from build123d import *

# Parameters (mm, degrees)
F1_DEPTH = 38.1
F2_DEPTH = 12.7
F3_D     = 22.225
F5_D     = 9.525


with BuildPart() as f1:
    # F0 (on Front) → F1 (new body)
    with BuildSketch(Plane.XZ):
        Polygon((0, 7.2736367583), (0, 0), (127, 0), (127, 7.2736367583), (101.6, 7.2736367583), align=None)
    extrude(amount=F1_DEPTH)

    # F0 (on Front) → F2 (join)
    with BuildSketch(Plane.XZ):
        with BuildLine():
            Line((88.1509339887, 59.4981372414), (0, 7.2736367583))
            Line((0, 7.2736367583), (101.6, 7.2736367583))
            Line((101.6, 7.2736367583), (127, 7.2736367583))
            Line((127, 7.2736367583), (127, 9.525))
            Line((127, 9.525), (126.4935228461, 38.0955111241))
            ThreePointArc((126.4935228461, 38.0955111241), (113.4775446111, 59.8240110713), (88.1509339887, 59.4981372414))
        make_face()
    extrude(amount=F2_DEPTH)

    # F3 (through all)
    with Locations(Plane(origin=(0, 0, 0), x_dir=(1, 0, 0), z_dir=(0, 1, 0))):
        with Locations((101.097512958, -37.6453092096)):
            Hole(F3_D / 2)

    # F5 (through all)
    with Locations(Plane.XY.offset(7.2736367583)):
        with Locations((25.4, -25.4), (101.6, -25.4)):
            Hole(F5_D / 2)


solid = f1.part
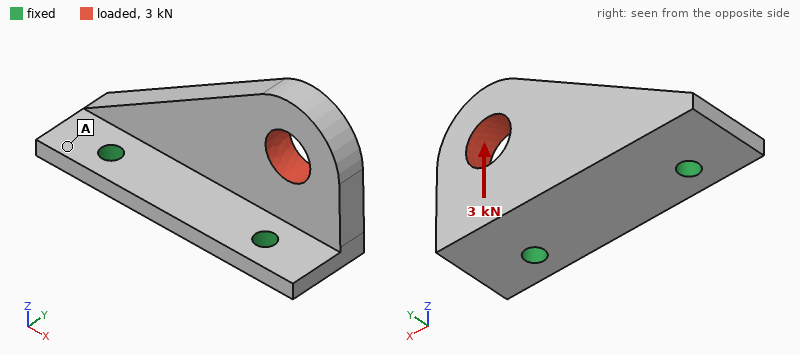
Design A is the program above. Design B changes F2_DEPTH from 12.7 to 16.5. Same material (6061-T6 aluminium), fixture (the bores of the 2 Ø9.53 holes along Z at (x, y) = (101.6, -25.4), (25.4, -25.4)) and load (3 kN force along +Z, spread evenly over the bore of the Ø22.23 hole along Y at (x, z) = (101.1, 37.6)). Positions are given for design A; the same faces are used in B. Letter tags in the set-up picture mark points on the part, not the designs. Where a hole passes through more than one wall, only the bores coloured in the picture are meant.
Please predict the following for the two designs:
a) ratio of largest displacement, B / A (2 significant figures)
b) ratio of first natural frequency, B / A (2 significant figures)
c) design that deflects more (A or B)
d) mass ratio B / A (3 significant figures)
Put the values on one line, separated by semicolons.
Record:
0.75; 1.0; A; 1.18
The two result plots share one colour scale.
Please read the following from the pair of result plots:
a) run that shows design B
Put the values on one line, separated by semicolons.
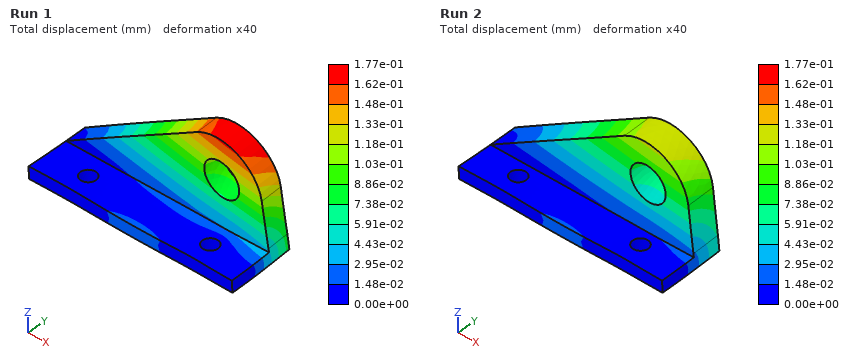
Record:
Run 2
